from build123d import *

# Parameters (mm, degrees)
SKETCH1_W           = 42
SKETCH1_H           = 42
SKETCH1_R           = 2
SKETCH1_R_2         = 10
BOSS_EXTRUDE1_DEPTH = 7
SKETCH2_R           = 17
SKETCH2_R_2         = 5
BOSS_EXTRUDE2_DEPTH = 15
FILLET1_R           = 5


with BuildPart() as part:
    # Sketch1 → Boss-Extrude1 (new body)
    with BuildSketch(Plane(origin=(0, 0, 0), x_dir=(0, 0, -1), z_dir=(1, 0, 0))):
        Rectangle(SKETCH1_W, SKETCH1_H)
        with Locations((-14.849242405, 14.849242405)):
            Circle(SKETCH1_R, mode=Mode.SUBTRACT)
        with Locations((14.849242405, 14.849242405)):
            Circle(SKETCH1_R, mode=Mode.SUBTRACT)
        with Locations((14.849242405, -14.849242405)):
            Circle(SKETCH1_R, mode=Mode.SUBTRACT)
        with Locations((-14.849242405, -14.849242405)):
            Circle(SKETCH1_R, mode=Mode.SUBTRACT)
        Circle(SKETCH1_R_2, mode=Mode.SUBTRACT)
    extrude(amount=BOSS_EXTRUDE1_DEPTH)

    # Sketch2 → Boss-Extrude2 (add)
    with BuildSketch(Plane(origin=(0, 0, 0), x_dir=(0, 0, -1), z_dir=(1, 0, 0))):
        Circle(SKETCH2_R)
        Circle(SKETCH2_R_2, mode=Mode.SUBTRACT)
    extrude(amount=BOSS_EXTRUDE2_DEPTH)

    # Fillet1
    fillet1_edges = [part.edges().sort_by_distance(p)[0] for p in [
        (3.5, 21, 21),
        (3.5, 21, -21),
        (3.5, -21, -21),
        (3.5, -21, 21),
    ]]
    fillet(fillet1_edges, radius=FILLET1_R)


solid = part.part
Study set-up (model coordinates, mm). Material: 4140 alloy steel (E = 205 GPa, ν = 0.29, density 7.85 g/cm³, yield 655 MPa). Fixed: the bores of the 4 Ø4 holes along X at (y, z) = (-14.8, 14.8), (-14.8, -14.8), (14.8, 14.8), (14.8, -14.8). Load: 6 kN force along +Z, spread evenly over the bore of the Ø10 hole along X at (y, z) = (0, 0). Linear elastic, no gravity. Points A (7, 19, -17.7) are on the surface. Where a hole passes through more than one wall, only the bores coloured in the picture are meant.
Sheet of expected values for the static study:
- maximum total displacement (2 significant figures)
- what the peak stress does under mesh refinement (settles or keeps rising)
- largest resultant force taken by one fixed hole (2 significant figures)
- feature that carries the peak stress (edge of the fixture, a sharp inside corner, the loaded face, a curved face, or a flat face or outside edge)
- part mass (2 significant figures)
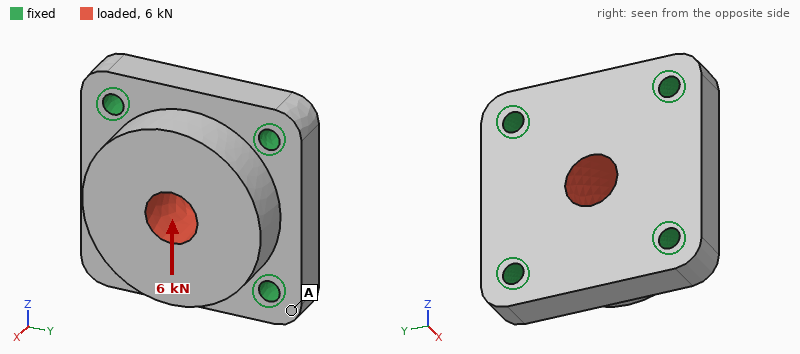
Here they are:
2.2 µm
keeps rising
1.7 kN
edge of the fixture
140 g
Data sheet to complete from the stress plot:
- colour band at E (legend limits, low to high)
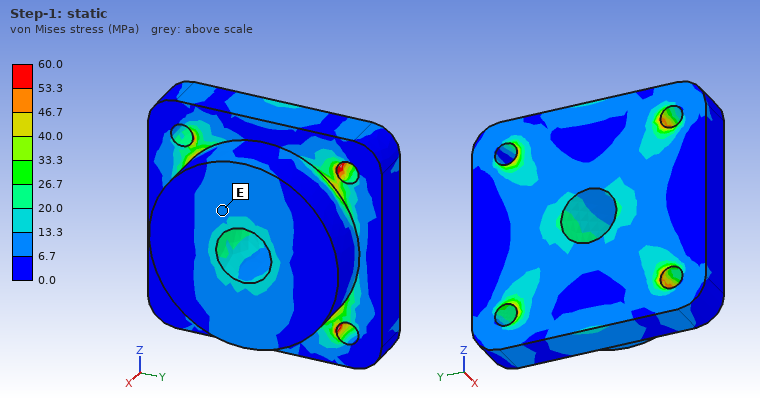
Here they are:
6.7 to 13.3 MPa
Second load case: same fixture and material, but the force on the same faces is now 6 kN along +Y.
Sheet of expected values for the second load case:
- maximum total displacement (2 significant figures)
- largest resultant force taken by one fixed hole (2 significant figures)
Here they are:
2.2 µm
1.7 kN
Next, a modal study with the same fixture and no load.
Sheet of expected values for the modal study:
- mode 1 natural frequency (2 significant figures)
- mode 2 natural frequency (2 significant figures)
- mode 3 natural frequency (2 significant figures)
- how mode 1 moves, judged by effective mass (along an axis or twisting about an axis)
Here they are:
25 kHz
31 kHz
31 kHz
along X
